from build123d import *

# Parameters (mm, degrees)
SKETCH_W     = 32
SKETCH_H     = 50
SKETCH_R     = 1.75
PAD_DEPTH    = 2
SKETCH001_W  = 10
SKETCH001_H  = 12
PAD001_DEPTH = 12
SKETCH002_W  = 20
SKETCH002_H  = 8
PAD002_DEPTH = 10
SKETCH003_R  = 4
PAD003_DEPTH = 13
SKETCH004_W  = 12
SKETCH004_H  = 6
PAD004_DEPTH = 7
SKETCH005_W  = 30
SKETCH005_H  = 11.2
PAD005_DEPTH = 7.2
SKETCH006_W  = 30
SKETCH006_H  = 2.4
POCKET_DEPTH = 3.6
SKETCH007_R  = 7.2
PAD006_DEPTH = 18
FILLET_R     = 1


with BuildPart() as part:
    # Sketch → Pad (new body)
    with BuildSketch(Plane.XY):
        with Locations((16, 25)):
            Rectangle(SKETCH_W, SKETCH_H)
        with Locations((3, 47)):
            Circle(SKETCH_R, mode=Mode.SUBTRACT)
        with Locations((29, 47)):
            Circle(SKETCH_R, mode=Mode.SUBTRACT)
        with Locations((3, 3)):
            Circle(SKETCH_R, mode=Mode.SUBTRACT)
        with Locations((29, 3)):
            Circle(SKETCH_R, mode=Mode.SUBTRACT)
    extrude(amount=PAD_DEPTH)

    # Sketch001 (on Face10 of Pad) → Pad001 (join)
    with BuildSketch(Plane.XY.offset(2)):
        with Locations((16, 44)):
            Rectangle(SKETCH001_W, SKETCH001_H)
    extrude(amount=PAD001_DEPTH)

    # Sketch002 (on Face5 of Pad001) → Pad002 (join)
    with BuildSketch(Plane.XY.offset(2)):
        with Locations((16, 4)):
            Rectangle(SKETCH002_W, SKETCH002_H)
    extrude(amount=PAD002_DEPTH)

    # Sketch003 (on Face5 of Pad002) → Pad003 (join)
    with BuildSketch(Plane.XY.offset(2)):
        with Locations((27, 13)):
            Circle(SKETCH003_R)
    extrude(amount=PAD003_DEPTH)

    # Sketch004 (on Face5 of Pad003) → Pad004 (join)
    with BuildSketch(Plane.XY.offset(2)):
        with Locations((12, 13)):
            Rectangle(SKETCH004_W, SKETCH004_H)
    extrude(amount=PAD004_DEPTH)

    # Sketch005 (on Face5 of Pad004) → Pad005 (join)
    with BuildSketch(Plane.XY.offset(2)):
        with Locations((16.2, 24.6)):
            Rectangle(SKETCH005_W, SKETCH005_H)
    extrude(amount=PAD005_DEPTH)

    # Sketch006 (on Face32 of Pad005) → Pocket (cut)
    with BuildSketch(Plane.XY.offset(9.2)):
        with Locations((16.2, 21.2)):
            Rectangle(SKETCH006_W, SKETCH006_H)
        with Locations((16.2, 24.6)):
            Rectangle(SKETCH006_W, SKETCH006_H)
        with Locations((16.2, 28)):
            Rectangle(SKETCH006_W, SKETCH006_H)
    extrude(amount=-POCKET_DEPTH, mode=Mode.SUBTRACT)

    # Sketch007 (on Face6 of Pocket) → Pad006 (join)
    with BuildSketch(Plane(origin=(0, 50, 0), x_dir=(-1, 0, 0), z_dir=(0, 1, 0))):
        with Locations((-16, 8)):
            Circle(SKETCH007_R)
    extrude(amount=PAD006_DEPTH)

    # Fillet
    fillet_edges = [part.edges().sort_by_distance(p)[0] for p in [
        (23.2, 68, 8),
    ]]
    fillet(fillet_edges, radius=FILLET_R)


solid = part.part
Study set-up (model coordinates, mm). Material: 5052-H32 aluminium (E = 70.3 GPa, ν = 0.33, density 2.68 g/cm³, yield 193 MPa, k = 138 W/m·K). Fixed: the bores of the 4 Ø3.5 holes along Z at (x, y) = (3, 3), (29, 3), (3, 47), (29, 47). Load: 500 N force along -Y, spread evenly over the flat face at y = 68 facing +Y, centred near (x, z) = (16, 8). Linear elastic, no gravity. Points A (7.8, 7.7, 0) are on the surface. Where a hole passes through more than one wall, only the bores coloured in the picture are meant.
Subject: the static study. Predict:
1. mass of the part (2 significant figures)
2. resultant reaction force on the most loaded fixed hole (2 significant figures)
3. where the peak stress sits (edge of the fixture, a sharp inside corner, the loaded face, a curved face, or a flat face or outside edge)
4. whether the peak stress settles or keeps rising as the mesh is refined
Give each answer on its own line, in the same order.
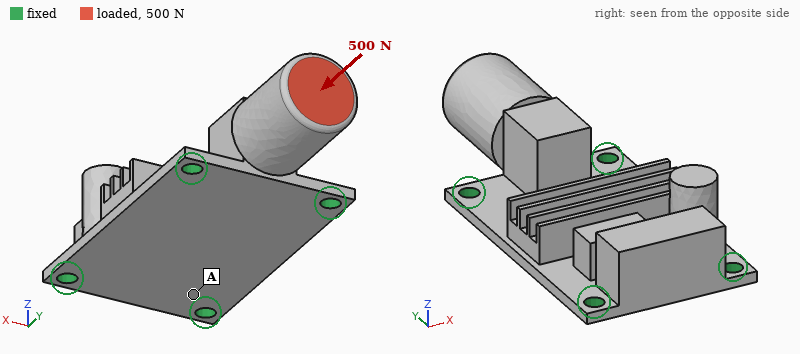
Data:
32 g
190 N
edge of the fixture
keeps rising
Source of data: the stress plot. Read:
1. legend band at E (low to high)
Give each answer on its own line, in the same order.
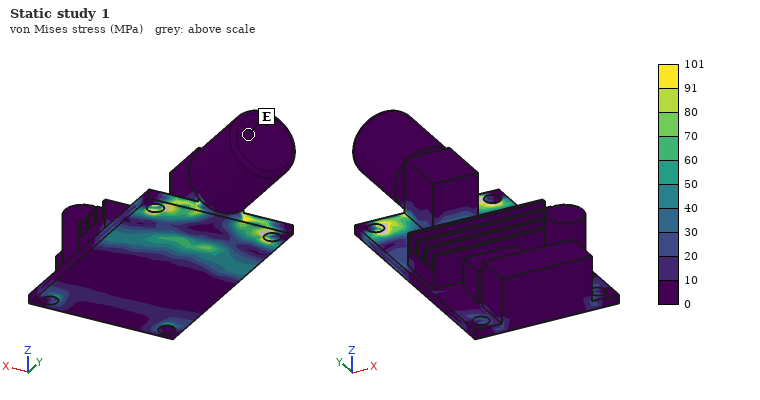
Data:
0 to 10 MPa
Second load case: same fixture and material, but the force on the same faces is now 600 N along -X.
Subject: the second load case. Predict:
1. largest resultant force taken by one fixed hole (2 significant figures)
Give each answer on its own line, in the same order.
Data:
550 N
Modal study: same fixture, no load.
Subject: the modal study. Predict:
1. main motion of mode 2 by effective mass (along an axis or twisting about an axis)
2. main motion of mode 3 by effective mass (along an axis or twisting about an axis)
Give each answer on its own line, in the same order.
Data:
along Z
along X
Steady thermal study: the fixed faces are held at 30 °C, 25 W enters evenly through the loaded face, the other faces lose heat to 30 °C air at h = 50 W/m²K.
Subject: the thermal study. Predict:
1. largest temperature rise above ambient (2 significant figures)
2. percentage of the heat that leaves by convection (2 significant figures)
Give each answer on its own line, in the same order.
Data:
54 K
18 %
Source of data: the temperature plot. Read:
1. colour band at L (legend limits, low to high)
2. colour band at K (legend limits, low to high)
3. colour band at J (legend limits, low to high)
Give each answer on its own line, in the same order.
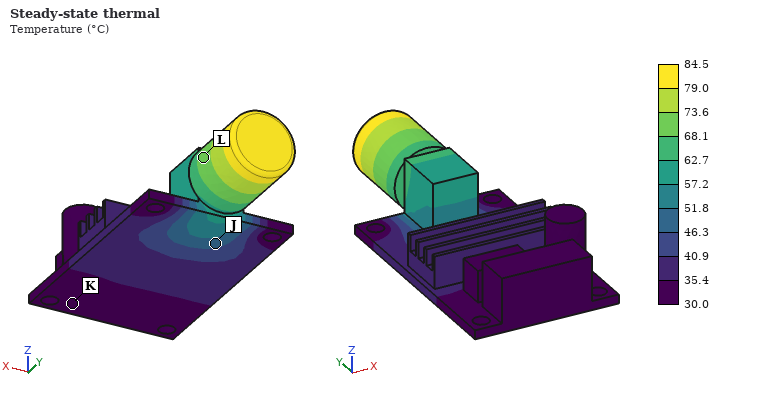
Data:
68.1 to 73.6 °C
30.0 to 35.4 °C
46.3 to 51.8 °C
